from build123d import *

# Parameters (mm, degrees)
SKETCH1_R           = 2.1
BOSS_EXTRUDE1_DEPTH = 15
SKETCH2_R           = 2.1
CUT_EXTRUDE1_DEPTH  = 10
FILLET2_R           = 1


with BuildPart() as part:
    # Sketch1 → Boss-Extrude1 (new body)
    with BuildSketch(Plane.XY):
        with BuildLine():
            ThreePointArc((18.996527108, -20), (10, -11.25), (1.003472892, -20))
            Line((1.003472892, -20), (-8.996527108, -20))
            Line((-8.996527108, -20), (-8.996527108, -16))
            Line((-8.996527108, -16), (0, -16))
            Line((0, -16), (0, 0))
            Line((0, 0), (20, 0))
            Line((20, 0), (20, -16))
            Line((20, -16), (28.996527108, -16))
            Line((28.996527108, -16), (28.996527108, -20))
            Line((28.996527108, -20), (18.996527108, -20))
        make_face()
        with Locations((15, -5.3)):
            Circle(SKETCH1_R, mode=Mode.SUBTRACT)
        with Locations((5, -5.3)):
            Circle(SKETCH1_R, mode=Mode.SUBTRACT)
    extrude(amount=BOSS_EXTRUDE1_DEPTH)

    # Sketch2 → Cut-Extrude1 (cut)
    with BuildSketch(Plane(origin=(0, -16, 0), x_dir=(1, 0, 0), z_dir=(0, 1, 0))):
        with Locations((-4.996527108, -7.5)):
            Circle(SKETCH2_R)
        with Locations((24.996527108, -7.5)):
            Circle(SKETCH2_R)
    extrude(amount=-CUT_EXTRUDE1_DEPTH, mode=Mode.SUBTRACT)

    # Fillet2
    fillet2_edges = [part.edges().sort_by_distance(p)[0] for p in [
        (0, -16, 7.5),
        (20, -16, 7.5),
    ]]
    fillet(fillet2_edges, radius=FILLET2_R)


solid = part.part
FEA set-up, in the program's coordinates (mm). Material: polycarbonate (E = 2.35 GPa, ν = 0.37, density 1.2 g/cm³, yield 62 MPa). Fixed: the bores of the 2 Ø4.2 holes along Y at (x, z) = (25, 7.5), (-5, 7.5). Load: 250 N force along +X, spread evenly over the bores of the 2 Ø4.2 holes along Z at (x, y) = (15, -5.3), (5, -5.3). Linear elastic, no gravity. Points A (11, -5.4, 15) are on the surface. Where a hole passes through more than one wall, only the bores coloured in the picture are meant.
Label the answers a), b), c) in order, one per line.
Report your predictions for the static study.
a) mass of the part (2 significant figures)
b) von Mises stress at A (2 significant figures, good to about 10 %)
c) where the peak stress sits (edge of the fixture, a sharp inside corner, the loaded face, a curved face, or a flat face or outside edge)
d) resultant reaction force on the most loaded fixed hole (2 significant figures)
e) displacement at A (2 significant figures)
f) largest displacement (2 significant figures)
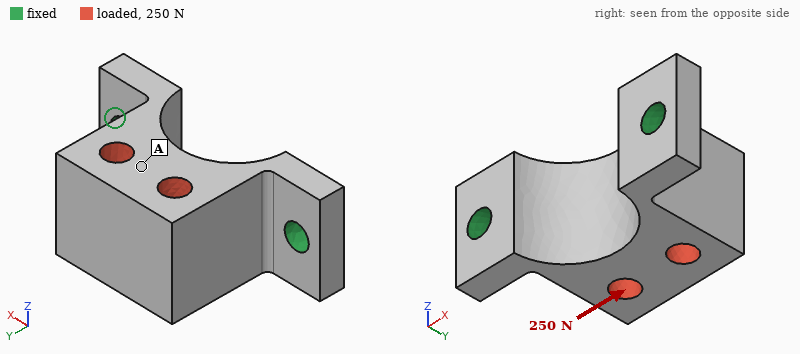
a) 5.7 g
b) 3.0 MPa
c) a curved face
d) 180 N
e) 63 µm
f) 88 µm
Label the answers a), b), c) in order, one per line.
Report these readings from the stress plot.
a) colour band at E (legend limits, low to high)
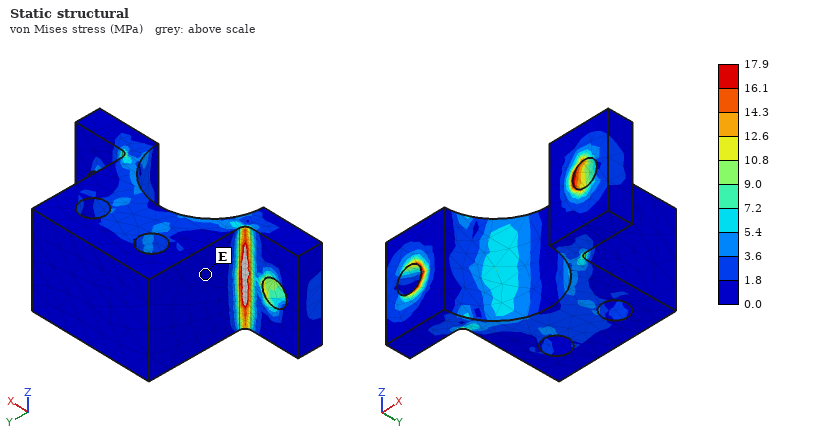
a) 0.0 to 1.8 MPa
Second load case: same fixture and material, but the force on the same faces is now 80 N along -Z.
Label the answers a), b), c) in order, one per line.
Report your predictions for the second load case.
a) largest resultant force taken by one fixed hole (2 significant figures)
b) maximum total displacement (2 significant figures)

a) 40 N
b) 0.22 mm
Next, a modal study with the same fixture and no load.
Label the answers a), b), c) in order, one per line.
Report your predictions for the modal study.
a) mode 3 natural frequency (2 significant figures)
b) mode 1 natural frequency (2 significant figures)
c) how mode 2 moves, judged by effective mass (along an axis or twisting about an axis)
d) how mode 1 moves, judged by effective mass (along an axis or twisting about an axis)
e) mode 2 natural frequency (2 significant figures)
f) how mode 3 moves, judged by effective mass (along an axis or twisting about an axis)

a) 5900 Hz
b) 1800 Hz
c) along X
d) along Z
e) 4800 Hz
f) along Y
